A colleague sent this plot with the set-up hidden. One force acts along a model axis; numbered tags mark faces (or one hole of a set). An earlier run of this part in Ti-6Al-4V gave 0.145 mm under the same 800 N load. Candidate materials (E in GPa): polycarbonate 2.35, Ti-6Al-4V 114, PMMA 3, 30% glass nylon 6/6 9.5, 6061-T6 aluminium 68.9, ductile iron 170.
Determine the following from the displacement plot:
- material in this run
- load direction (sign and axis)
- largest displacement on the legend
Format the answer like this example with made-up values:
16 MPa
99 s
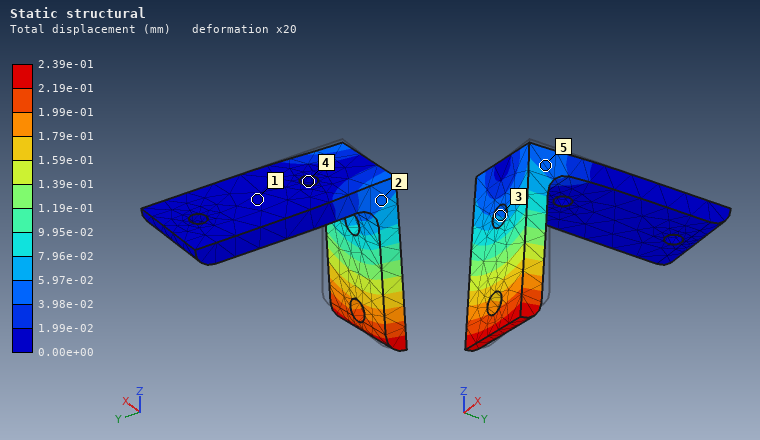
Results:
6061-T6 aluminium
-X
2.39e-01 mm
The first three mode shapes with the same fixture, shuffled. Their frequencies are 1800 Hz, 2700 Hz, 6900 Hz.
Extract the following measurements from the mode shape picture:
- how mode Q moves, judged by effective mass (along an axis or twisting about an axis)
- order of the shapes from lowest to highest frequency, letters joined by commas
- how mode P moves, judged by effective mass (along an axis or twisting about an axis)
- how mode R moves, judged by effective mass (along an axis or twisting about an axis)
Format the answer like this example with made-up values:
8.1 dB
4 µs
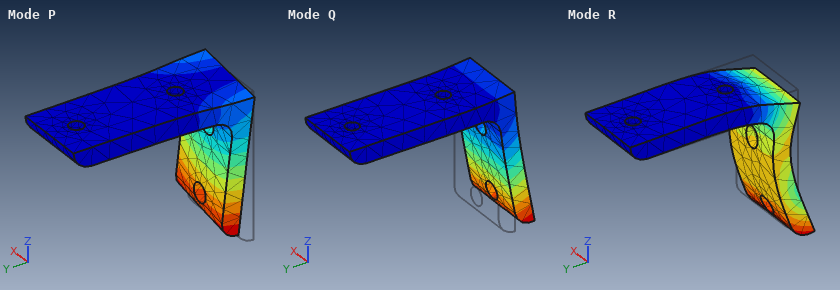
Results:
along Y
Q, P, R
along X
along Z
